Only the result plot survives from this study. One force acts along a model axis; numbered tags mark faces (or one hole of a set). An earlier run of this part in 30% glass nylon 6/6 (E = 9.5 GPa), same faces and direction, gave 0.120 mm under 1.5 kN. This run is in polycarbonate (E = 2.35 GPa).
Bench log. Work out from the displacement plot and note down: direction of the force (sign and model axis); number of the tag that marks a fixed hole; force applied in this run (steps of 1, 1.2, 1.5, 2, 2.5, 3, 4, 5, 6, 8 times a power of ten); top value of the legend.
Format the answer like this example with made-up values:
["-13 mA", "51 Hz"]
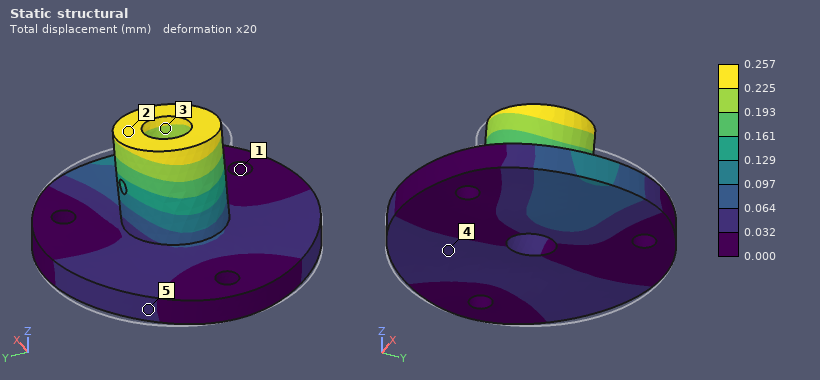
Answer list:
["+X", "1", "800 N", "0.257 mm"]
